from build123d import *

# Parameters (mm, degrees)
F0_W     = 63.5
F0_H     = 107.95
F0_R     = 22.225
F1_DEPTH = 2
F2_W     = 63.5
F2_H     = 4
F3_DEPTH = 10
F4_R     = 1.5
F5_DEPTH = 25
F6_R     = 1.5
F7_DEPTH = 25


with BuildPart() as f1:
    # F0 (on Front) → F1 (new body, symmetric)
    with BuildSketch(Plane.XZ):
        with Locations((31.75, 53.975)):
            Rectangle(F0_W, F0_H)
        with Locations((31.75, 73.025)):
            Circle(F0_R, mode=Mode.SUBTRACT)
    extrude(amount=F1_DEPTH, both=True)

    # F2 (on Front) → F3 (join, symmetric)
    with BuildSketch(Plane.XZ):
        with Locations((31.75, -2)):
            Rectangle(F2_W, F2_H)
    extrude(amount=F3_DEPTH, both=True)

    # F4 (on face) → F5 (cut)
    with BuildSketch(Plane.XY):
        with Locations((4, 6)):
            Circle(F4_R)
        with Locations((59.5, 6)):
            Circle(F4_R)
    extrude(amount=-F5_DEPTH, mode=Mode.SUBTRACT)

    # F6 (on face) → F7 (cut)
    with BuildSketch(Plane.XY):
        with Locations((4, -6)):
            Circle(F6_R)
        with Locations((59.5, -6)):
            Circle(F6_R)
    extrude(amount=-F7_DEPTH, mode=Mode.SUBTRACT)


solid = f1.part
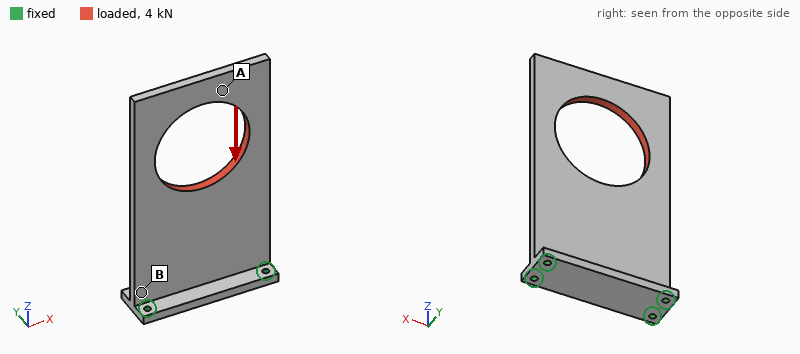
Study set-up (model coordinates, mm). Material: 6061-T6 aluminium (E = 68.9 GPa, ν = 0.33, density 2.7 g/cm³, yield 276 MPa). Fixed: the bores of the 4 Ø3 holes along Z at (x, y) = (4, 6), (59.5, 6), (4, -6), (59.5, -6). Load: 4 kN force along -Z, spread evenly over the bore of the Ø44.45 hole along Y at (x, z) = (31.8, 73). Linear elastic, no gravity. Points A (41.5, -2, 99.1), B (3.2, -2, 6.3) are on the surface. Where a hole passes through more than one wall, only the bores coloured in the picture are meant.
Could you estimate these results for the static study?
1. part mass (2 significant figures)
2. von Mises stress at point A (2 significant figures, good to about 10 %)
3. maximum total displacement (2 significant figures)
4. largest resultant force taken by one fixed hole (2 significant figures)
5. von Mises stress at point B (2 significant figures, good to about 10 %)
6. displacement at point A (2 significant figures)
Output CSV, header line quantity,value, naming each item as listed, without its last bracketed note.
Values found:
quantity,value
part mass,71 g
von Mises stress at point A,14 MPa
maximum total displacement,69 µm
largest resultant force taken by one fixed hole,1.1 kN
von Mises stress at point B,37 MPa
displacement at point A,64 µm
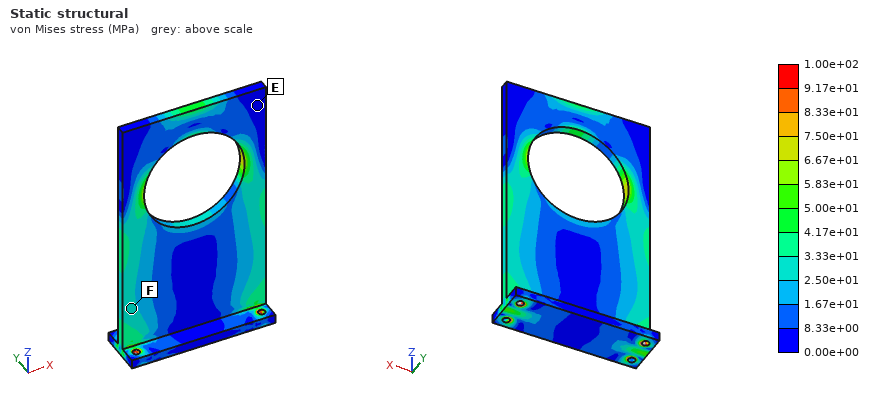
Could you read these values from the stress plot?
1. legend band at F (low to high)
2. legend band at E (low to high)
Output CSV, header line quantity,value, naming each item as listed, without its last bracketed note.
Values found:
quantity,value
legend band at F,2.50e+01 to 3.33e+01 MPa
legend band at E,0.00e+00 to 8.33e+00 MPa
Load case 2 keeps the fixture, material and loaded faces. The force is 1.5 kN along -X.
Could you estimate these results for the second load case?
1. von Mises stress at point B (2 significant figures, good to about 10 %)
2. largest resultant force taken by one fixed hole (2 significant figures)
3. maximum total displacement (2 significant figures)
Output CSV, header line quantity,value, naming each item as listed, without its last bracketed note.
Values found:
quantity,value
von Mises stress at point B,42 MPa
largest resultant force taken by one fixed hole,1.1 kN
maximum total displacement,0.19 mm
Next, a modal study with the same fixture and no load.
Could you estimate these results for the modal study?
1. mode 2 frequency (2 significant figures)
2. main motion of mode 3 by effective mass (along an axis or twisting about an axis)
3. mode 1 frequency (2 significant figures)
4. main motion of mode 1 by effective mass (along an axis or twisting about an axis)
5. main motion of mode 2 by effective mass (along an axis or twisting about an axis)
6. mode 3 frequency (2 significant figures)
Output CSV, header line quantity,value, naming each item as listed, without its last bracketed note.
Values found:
quantity,value
mode 2 frequency,930 Hz
main motion of mode 3 by effective mass,along Y
mode 1 frequency,290 Hz
main motion of mode 1 by effective mass,along Y
main motion of mode 2 by effective mass,twisting about Z
mode 3 frequency,1400 Hz
